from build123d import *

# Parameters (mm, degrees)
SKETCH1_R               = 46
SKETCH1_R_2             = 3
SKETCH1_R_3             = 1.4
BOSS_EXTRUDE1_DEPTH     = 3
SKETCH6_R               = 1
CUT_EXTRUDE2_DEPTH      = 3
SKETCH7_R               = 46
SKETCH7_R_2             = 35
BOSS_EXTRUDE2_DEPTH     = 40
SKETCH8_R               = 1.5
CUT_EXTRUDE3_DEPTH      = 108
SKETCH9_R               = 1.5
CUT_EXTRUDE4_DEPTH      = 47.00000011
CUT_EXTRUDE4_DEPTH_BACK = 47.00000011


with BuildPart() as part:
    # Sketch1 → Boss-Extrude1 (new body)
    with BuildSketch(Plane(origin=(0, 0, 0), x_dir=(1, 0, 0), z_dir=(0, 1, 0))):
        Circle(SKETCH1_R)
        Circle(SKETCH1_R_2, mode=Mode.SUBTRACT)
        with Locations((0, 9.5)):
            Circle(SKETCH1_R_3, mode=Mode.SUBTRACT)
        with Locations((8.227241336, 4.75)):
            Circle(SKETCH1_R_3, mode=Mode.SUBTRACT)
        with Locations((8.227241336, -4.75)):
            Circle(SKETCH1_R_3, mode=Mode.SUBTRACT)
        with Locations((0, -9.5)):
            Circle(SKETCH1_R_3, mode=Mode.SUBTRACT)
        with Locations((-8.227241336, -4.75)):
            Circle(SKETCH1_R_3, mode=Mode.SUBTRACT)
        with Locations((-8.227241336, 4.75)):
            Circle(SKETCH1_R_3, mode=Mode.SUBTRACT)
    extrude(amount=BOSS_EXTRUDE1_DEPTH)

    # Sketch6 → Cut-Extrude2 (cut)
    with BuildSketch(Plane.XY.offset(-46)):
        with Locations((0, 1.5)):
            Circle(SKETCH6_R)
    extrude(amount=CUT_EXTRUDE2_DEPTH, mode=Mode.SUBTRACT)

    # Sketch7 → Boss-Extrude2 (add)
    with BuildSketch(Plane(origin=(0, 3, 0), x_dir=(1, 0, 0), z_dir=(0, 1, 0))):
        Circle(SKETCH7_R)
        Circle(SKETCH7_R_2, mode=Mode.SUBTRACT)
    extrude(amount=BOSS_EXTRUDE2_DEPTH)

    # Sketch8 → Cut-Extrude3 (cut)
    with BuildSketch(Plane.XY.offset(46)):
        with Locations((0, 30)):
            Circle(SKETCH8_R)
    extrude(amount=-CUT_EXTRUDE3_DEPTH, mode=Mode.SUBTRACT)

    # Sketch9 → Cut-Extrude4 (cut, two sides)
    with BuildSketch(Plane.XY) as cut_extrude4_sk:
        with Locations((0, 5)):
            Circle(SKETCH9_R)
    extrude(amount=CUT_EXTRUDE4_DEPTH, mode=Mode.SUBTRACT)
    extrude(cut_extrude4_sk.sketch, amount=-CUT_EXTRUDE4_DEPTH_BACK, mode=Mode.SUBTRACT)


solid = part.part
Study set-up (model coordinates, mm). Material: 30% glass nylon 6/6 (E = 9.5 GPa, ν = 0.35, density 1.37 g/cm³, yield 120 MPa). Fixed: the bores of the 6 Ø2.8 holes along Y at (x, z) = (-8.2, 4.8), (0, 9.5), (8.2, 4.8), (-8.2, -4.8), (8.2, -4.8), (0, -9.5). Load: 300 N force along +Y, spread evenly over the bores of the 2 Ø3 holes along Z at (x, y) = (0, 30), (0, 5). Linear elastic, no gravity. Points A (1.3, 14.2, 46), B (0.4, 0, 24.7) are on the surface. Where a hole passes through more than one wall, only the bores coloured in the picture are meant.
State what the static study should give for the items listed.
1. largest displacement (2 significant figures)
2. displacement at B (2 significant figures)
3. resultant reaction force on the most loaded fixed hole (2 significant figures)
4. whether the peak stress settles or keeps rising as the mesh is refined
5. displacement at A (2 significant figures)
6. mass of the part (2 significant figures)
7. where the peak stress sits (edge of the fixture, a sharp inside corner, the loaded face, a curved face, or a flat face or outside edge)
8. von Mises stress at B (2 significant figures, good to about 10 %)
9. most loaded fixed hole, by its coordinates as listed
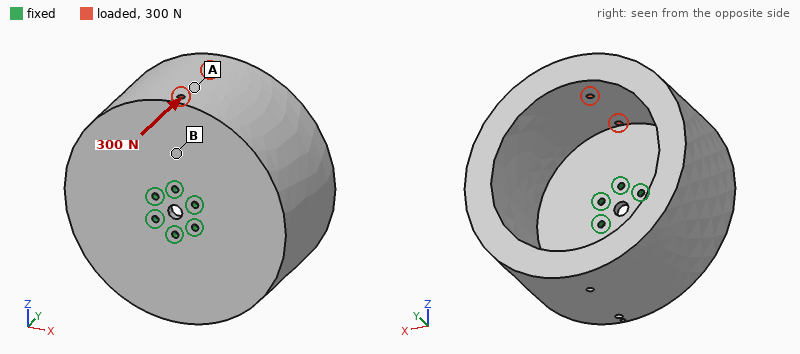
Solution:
1.3 mm
0.47 mm
280 N
keeps rising
1.1 mm
180 g
edge of the fixture
16 MPa
(0, 9.5)
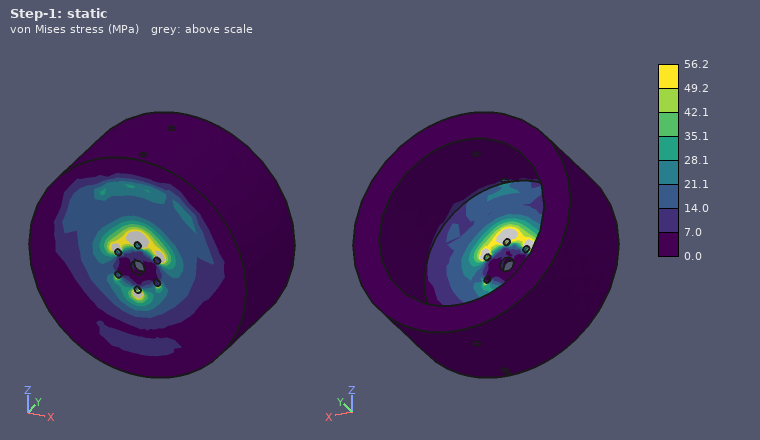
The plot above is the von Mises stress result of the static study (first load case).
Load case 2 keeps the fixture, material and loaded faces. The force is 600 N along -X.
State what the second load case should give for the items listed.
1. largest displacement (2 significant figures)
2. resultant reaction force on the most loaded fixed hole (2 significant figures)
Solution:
0.98 mm
540 N
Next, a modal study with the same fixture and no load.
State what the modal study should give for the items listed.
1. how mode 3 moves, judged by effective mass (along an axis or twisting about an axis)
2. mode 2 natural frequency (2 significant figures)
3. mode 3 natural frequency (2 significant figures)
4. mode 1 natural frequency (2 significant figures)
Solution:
along Y
260 Hz
570 Hz
260 Hz
